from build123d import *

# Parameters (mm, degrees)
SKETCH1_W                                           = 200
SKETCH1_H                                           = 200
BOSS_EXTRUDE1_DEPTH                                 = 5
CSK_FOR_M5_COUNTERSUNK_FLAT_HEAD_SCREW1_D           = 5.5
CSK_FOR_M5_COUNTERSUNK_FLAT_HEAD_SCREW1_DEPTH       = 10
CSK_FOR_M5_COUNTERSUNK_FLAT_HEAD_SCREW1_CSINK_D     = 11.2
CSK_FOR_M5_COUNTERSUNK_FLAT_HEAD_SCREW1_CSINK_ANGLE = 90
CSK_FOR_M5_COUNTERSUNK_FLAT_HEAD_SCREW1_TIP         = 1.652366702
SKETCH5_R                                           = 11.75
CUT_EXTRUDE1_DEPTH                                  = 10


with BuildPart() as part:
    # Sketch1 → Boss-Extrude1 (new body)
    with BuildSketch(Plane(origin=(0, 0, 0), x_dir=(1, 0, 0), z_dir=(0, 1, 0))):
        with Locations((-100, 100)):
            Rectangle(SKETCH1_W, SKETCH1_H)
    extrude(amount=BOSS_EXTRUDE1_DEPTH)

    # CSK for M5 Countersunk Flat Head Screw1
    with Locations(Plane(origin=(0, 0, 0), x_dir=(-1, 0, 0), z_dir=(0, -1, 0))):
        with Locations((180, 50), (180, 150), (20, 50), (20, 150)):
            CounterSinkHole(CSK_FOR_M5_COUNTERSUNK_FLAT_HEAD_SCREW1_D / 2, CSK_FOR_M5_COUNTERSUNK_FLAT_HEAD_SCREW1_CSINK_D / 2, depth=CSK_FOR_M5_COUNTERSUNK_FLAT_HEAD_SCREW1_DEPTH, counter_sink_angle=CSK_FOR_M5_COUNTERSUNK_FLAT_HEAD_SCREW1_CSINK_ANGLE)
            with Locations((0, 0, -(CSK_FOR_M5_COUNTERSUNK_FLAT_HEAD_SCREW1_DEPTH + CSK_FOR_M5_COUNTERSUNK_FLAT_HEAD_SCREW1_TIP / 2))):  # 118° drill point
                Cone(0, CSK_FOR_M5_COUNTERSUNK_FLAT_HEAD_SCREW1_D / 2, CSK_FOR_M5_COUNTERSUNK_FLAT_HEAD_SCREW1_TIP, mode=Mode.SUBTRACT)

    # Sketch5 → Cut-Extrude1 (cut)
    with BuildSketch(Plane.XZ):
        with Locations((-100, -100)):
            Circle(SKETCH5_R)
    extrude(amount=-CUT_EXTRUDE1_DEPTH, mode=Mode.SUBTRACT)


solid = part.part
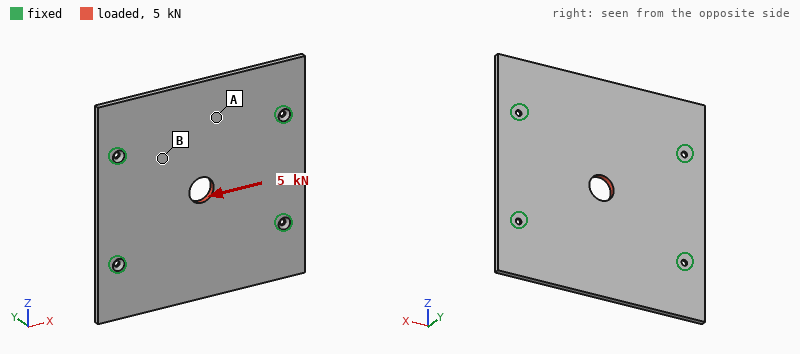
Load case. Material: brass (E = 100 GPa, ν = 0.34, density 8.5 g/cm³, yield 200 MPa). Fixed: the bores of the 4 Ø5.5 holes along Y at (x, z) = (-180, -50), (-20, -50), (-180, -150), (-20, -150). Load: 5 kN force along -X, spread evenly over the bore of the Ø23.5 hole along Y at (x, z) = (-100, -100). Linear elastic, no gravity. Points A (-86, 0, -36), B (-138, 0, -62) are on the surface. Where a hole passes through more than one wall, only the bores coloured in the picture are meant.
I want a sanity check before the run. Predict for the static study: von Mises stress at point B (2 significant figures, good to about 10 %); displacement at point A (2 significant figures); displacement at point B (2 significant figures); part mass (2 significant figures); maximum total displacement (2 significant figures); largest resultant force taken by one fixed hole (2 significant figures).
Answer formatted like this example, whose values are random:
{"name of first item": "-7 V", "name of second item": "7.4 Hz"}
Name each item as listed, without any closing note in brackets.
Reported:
{"von Mises stress at point B": "4.6 MPa", "displacement at point A": "3.0 µm", "displacement at point B": "5.2 µm", "part mass": "1.7 kg", "maximum total displacement": "8.7 µm", "largest resultant force taken by one fixed hole": "1.3 kN"}
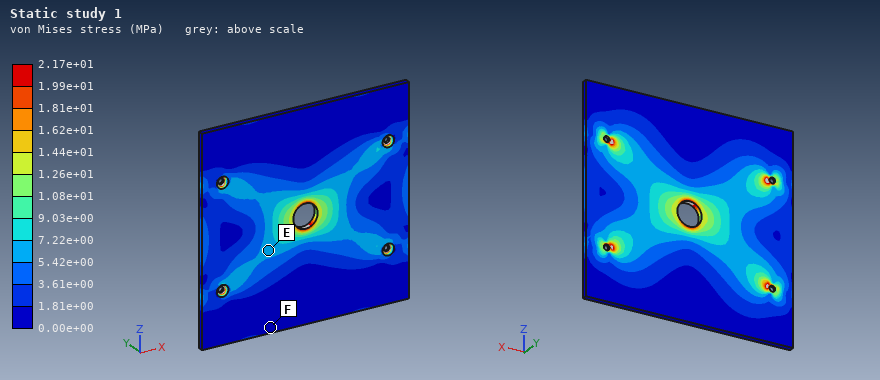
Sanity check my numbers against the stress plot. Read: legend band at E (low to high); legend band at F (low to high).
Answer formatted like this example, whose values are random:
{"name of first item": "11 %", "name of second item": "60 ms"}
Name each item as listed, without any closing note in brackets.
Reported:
{"legend band at E": "5.42e+00 to 7.22e+00 MPa", "legend band at F": "0.00e+00 to 1.81e+00 MPa"}
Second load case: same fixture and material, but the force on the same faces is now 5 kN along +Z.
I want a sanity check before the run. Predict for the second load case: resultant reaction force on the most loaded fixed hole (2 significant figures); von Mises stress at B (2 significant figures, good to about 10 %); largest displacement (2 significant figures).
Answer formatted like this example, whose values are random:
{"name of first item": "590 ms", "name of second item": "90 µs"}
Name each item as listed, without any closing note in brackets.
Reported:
{"resultant reaction force on the most loaded fixed hole": "1.3 kN", "von Mises stress at B": "5.6 MPa", "largest displacement": "12 µm"}
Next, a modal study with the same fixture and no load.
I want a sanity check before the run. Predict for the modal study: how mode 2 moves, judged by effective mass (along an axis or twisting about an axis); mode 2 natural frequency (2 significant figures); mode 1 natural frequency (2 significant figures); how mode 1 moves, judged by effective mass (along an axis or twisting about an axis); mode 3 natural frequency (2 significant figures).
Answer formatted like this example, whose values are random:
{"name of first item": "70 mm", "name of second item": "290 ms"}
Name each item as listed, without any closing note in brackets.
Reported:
{"how mode 2 moves, judged by effective mass": "twisting about X", "mode 2 natural frequency": "480 Hz", "mode 1 natural frequency": "440 Hz", "how mode 1 moves, judged by effective mass": "along Y", "mode 3 natural frequency": "650 Hz"}
